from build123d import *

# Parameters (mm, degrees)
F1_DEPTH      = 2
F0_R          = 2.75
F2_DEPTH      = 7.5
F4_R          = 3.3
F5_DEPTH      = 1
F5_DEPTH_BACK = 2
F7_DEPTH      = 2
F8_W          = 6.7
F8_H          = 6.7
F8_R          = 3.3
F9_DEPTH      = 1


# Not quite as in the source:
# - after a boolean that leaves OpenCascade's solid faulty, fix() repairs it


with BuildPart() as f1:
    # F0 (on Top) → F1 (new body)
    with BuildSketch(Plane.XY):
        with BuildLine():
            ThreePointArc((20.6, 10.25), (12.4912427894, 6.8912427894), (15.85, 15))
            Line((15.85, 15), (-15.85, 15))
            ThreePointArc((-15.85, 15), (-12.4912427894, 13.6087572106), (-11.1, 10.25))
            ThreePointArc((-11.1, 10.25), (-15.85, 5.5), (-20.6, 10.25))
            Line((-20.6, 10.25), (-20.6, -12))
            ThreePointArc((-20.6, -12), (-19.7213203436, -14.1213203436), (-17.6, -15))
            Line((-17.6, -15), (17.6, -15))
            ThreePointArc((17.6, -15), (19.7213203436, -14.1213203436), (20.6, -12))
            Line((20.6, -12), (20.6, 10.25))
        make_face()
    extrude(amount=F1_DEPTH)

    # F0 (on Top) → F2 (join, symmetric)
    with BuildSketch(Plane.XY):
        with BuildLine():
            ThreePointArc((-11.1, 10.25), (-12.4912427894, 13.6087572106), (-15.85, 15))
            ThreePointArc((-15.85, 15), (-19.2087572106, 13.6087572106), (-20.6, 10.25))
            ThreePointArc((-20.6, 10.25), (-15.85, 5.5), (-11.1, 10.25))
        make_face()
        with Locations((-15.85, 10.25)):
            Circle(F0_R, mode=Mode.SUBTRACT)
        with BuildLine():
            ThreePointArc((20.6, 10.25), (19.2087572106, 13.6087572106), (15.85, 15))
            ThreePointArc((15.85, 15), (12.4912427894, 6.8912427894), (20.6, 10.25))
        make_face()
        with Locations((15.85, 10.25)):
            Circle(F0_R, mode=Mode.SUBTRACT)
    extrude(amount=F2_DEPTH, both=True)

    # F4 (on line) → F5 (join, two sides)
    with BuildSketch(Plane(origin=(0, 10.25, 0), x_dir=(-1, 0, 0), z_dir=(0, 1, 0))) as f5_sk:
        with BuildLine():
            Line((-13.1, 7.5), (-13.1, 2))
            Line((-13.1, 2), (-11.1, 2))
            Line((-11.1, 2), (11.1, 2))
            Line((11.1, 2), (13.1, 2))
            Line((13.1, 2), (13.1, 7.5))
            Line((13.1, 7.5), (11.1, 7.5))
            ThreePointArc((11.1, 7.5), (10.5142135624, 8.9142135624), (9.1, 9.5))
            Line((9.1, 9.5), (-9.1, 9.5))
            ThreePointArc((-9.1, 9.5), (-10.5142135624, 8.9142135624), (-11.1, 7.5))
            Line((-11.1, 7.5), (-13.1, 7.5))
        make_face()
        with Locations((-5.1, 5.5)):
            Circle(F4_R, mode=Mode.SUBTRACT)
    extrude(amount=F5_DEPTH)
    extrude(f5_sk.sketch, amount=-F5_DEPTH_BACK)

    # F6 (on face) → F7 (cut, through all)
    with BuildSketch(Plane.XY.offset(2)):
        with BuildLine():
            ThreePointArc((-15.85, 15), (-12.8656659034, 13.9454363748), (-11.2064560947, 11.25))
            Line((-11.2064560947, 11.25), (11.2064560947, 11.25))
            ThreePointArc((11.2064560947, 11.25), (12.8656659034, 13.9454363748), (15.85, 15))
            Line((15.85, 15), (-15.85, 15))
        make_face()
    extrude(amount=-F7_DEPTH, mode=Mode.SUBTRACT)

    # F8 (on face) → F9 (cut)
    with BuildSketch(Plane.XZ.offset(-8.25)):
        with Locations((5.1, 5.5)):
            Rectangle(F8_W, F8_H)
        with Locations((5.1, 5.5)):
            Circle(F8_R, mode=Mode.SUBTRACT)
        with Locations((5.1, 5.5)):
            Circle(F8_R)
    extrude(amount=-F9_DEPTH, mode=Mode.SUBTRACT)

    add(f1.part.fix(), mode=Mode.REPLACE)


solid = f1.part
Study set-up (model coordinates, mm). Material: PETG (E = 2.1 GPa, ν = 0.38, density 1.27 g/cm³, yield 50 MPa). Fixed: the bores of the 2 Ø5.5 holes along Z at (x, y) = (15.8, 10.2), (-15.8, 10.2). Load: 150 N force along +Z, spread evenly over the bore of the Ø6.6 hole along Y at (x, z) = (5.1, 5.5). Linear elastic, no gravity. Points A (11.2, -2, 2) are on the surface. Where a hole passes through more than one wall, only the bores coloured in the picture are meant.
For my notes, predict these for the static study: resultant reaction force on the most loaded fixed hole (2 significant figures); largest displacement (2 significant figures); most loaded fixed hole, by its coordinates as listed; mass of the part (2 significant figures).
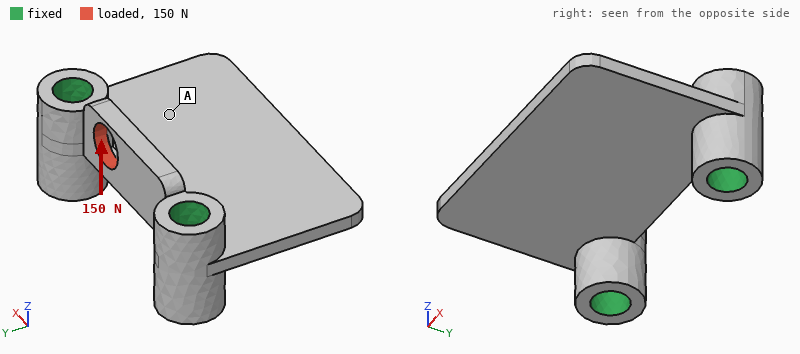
99 N
0.15 mm
(15.8, 10.2)
4.8 g
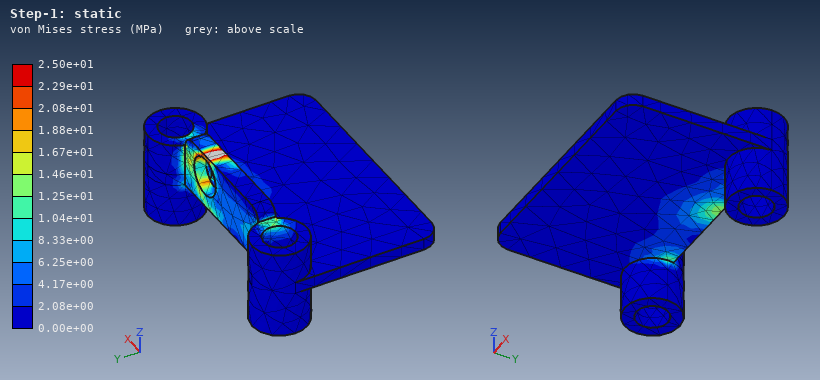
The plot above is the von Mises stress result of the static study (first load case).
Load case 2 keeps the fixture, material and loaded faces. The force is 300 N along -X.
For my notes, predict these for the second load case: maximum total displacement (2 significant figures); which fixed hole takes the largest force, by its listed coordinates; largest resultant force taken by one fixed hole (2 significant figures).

74 µm
(15.8, 10.2)
180 N
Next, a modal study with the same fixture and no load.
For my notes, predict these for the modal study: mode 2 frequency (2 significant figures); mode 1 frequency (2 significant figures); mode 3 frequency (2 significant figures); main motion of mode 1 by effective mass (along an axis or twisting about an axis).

1400 Hz
830 Hz
2700 Hz
along Z
